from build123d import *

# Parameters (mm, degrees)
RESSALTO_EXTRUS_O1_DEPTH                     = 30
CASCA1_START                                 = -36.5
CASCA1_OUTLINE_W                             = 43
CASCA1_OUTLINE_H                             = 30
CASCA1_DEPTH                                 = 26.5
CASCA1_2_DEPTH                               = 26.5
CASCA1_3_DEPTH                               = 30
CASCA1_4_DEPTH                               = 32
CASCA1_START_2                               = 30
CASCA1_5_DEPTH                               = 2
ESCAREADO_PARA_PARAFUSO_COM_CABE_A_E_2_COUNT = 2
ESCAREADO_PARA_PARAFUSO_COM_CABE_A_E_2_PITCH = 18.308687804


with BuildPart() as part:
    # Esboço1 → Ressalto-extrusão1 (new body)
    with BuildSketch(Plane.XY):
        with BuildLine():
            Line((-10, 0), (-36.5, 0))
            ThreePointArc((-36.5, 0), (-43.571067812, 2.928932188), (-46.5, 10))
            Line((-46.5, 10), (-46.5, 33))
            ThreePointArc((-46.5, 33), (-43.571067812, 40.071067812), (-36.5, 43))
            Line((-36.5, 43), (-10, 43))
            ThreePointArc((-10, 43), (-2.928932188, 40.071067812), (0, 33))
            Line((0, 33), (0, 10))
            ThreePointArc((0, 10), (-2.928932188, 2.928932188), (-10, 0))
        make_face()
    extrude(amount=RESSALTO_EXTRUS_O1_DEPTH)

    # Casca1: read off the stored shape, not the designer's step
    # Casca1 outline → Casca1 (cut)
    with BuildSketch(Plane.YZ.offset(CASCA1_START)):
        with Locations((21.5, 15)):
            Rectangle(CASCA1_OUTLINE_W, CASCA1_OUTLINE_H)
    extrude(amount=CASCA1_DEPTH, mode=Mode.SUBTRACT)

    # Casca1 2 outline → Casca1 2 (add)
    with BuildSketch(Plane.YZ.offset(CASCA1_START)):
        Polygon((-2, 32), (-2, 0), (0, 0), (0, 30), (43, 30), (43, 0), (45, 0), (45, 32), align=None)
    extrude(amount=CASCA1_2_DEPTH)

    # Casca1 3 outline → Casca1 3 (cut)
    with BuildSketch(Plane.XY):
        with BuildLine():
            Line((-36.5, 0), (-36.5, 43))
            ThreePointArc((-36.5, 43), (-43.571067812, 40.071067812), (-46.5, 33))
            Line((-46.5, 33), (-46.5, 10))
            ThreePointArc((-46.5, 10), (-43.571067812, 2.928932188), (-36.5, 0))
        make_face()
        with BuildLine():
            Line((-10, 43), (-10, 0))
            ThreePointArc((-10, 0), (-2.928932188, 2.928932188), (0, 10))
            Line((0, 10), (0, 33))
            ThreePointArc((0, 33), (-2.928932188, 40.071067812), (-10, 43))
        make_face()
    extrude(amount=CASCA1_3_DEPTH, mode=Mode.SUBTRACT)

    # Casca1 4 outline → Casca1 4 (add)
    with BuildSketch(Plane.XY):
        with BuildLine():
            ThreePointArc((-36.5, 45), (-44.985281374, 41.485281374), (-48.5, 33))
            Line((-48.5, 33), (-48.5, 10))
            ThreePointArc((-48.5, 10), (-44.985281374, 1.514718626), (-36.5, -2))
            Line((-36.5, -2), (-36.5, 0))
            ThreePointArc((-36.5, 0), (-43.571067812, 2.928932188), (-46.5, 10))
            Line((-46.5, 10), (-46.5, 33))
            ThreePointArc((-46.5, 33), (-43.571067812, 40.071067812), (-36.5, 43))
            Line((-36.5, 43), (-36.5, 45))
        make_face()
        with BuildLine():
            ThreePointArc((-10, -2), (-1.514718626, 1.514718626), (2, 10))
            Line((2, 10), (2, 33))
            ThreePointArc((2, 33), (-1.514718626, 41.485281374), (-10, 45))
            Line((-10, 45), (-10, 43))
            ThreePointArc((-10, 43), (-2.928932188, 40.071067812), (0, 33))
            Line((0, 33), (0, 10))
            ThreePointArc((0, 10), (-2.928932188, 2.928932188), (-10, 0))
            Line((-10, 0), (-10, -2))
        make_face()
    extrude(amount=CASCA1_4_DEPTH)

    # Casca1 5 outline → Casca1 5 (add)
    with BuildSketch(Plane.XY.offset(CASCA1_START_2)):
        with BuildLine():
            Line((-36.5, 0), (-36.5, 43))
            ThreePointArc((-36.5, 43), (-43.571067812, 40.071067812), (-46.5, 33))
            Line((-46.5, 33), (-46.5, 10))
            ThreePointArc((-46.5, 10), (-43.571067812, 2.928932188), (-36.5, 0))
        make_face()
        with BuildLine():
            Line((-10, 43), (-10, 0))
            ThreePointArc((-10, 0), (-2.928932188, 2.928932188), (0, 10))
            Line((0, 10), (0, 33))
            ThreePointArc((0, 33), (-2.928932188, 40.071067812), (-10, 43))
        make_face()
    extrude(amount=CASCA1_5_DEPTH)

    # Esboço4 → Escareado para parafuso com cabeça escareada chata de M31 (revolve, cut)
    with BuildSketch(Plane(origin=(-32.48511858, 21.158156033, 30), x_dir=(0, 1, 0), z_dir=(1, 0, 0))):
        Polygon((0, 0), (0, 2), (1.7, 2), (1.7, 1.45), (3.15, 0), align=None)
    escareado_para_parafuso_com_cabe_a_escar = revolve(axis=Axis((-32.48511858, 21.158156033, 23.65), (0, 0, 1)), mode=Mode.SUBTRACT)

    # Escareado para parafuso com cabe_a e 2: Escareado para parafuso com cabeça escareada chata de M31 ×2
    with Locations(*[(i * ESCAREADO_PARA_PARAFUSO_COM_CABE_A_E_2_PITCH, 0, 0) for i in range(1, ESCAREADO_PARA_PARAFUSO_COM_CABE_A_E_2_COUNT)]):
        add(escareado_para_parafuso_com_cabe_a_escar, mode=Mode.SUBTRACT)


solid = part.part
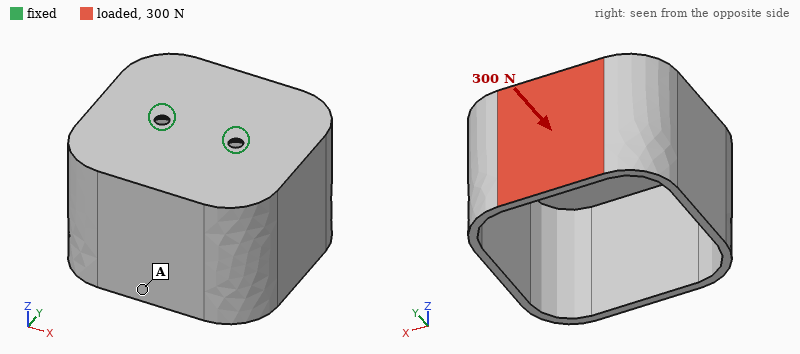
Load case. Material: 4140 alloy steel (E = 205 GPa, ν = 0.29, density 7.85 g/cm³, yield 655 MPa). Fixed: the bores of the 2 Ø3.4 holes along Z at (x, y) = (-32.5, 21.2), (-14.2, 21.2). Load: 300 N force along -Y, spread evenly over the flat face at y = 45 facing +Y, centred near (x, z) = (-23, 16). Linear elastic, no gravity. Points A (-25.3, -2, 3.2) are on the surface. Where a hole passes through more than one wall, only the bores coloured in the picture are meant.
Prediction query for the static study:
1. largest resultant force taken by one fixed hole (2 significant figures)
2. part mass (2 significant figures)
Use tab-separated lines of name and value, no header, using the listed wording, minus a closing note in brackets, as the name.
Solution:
largest resultant force taken by one fixed hole	160 N
part mass	110 g
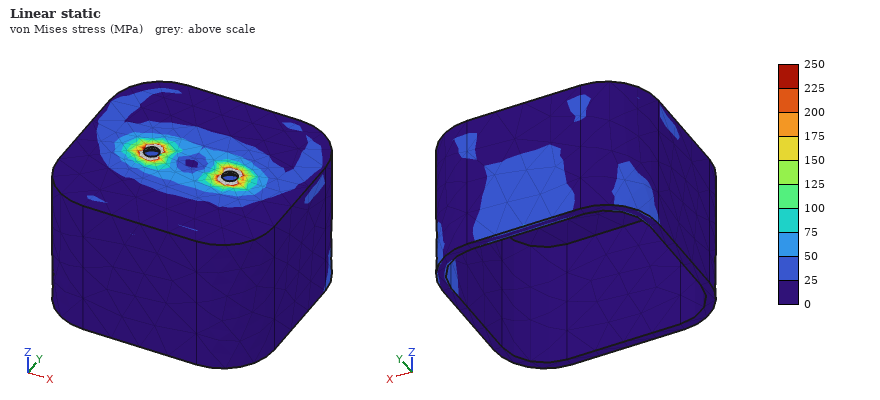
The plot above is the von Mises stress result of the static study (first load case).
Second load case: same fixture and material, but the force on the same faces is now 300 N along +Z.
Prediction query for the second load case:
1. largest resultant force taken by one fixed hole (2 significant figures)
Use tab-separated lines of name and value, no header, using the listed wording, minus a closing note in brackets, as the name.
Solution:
largest resultant force taken by one fixed hole	240 N
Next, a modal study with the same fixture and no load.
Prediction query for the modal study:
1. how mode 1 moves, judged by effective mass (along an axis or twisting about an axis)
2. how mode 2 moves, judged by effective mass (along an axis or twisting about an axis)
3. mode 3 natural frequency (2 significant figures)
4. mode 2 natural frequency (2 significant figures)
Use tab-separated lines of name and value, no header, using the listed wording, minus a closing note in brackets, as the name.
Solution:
how mode 1 moves, judged by effective mass	along Y
how mode 2 moves, judged by effective mass	along X
mode 3 natural frequency	2100 Hz
mode 2 natural frequency	1200 Hz
